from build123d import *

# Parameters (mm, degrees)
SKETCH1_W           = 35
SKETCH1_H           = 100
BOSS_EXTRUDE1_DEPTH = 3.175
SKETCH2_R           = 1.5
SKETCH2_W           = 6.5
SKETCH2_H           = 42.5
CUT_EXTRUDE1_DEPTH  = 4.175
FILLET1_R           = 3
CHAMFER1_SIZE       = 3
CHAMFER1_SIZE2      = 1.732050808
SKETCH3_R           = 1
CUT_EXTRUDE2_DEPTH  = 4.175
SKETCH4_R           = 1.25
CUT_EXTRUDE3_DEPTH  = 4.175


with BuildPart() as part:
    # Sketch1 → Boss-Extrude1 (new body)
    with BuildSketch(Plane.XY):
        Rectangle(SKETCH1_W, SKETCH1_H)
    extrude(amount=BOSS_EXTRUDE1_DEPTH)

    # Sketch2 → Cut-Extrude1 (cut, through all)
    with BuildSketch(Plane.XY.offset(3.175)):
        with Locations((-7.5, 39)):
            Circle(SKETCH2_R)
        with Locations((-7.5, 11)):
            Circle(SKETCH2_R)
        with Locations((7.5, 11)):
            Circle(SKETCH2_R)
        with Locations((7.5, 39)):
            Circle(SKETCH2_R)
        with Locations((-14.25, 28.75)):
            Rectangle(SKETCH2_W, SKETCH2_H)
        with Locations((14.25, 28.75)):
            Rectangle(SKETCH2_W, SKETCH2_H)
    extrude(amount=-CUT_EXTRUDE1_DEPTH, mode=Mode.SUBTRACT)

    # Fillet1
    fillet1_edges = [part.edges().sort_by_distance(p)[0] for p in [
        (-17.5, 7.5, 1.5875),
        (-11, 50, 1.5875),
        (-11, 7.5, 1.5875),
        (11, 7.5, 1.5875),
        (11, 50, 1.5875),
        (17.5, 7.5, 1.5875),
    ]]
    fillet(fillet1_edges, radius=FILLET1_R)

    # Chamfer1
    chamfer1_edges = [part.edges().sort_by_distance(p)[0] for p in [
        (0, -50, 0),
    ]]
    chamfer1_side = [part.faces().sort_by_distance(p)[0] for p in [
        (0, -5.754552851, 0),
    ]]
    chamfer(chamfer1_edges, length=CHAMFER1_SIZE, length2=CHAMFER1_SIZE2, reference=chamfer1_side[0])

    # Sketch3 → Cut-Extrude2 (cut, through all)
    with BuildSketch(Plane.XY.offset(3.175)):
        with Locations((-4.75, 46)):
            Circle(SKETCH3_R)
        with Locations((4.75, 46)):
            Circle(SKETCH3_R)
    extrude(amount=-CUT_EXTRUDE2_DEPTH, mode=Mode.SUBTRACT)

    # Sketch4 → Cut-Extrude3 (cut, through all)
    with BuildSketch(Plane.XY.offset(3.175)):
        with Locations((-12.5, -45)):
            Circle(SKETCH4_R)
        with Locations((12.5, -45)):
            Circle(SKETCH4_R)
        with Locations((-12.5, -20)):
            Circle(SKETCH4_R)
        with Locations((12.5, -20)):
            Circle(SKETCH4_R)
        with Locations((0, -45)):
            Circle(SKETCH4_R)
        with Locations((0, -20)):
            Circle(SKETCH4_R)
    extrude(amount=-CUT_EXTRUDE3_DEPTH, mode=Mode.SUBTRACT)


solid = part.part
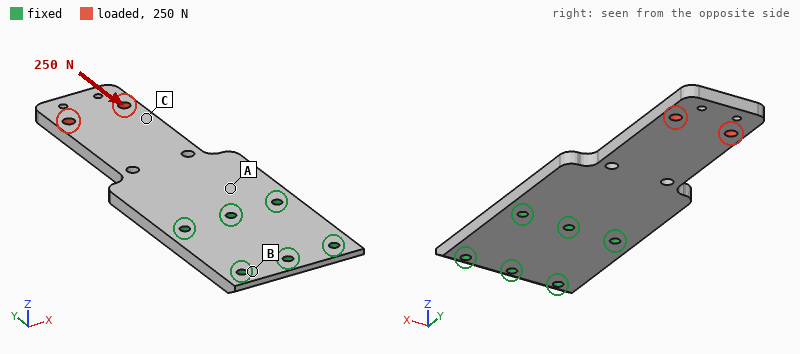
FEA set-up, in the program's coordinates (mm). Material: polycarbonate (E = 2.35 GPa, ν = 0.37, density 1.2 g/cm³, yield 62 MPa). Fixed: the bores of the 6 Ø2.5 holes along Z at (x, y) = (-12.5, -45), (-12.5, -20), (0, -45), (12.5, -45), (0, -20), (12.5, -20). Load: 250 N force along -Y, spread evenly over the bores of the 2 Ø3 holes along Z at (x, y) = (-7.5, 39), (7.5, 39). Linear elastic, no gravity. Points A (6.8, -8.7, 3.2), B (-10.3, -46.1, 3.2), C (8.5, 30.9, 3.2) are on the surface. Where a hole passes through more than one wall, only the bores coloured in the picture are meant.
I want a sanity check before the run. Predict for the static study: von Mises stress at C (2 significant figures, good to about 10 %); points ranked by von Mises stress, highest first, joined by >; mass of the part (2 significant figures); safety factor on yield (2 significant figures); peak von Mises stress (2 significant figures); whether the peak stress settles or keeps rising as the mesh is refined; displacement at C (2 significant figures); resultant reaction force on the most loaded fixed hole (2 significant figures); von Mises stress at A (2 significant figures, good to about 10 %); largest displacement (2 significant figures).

3.9 MPa
C > A > B
11 g
5.0
12 MPa
settles
70 µm
78 N
2.5 MPa
90 µm
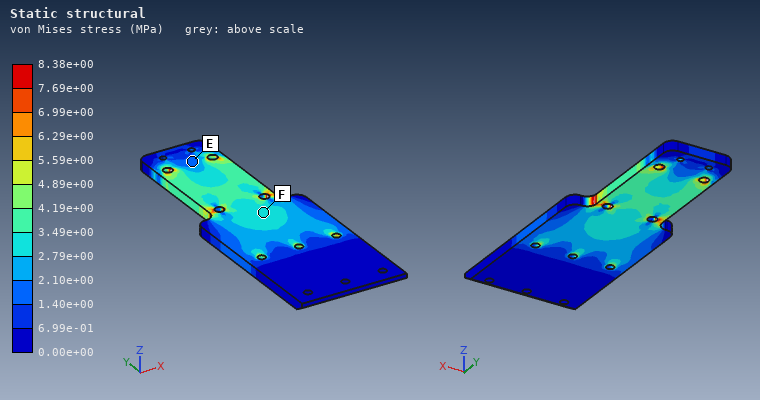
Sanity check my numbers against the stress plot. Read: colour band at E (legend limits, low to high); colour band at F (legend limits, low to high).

1.40e+00 to 2.10e+00 MPa
2.79e+00 to 3.49e+00 MPa
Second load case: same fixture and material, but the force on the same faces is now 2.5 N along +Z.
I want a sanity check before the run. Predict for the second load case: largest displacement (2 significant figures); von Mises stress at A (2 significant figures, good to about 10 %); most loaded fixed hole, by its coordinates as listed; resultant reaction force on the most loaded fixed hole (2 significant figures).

1.1 mm
1.9 MPa
(0, -20)
3.7 N
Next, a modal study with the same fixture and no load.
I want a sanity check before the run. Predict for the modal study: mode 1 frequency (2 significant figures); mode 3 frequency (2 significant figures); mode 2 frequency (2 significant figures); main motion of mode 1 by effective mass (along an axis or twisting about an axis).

180 Hz
1000 Hz
940 Hz
along Z
